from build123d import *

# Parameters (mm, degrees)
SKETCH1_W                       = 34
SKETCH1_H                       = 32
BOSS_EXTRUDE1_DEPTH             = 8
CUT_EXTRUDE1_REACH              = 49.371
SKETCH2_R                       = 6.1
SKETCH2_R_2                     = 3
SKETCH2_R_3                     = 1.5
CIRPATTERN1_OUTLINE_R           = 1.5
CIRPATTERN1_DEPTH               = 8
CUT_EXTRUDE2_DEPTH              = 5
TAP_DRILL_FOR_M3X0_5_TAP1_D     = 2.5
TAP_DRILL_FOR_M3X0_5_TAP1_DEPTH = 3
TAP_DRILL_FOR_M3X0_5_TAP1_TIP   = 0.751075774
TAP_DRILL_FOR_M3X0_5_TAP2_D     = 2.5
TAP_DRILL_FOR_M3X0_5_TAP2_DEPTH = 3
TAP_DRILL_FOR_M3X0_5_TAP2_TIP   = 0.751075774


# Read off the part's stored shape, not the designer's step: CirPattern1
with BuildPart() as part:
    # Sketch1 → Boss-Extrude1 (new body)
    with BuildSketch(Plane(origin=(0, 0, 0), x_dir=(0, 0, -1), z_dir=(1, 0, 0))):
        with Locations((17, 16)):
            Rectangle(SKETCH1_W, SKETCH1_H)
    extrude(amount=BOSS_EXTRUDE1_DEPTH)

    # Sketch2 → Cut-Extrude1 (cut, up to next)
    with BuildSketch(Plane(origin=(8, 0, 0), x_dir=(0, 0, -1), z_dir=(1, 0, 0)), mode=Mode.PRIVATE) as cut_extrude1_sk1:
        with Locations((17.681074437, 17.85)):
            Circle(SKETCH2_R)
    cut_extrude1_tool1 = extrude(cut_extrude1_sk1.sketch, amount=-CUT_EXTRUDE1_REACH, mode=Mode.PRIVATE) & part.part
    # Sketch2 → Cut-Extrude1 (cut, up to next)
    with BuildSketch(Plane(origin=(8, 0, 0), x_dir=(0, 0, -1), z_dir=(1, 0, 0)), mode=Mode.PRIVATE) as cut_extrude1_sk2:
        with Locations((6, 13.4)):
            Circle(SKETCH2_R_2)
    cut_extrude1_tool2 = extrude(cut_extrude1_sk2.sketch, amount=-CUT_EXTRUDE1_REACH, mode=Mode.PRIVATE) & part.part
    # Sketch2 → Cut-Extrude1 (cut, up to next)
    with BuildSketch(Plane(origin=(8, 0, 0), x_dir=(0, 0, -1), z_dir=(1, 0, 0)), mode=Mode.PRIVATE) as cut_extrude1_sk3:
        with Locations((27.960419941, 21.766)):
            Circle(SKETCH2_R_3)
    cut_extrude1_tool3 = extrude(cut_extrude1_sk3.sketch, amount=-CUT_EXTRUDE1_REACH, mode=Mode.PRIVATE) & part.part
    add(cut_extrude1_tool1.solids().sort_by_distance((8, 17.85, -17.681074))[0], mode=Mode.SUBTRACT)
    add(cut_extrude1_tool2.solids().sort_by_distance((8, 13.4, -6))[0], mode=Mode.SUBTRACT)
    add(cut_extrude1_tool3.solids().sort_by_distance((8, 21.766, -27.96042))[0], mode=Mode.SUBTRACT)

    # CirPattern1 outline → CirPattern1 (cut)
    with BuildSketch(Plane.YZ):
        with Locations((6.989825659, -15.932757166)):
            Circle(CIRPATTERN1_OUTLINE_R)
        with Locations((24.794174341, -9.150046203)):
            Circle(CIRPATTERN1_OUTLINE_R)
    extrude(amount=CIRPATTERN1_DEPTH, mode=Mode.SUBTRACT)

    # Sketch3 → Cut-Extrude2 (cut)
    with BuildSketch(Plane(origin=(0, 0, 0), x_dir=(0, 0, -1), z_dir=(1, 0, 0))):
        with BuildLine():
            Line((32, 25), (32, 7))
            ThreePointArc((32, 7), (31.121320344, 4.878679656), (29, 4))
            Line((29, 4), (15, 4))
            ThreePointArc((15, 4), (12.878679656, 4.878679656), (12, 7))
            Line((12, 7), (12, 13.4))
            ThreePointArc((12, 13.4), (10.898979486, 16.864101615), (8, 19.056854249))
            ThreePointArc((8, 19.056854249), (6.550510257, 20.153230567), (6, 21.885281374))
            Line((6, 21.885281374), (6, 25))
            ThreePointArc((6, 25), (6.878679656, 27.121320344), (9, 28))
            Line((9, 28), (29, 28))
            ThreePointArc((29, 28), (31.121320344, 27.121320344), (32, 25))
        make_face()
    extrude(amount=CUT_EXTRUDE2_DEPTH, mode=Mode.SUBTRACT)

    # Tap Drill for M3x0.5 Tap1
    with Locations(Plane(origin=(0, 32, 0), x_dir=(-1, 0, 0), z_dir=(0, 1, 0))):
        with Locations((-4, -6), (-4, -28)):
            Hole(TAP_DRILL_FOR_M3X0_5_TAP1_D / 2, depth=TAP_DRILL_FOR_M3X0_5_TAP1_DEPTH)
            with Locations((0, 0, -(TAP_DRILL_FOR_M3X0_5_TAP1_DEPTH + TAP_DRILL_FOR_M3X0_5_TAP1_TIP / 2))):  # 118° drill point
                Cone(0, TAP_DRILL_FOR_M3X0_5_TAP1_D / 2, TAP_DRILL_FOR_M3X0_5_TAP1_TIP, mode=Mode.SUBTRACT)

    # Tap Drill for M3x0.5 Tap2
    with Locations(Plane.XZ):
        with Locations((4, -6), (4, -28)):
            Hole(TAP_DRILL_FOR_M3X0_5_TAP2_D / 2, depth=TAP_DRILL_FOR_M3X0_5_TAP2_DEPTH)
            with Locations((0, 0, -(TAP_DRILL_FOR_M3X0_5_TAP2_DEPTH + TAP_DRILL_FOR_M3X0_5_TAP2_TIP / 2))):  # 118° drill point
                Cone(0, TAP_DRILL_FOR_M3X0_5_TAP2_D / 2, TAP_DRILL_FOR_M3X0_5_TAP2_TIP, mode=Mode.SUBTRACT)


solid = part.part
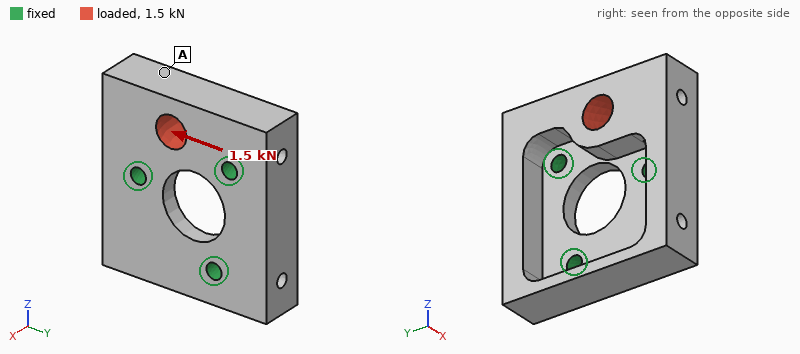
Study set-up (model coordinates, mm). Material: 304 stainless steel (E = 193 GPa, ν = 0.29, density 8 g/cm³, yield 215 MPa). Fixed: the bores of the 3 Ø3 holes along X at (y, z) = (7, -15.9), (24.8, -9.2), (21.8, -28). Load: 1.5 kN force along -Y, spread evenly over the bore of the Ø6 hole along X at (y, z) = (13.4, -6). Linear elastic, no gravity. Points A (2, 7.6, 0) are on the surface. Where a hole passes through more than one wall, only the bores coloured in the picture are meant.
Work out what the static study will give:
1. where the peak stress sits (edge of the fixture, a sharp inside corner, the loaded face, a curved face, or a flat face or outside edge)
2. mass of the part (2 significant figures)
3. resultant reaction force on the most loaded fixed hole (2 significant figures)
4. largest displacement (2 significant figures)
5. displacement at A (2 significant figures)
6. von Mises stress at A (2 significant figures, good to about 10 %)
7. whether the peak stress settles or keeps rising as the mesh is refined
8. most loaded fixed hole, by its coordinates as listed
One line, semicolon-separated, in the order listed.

edge of the fixture; 43 g; 1.1 kN; 5.3 µm; 4.3 µm; 11 MPa; keeps rising; (24.8, -9.2)
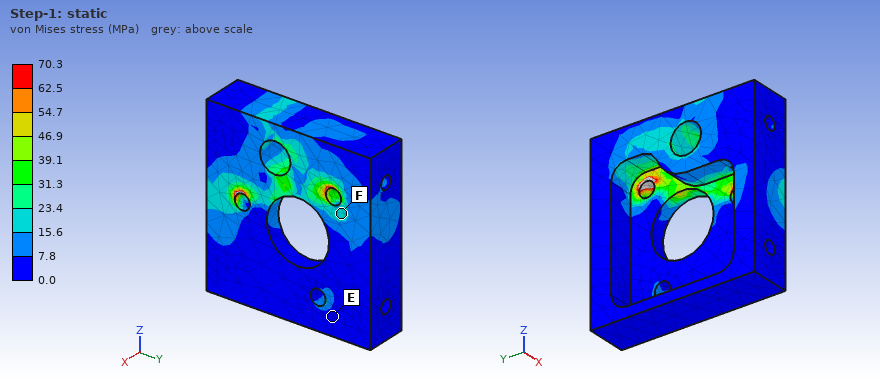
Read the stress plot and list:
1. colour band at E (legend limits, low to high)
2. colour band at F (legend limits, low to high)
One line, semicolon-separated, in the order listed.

0.0 to 7.8 MPa; 15.6 to 23.4 MPa
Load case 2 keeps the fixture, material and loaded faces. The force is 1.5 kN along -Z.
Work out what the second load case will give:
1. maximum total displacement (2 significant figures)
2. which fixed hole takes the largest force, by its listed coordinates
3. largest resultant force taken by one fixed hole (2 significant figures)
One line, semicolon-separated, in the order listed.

9.6 µm; (7, -15.9); 1.0 kN
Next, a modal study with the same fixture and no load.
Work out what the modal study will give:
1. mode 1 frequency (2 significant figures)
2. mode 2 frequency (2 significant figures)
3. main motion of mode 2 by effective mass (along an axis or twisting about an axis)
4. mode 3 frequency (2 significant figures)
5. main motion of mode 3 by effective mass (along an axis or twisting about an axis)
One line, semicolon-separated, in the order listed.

9600 Hz; 14 kHz; along X; 20 kHz; along X
